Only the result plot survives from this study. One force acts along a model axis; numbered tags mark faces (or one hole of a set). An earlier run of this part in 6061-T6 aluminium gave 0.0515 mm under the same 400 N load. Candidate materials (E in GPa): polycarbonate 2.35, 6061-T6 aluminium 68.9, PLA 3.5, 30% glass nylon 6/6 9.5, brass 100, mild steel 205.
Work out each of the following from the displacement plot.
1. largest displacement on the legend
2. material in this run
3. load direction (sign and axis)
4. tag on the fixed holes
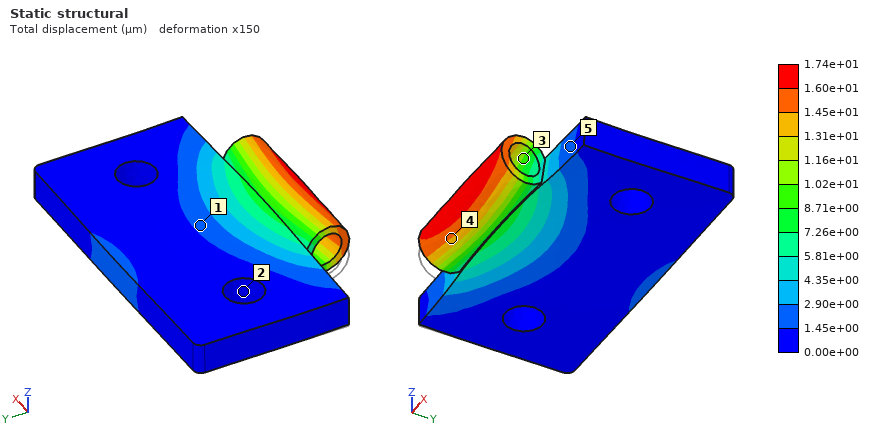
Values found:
1.74e+01 µm
mild steel
+Z
2
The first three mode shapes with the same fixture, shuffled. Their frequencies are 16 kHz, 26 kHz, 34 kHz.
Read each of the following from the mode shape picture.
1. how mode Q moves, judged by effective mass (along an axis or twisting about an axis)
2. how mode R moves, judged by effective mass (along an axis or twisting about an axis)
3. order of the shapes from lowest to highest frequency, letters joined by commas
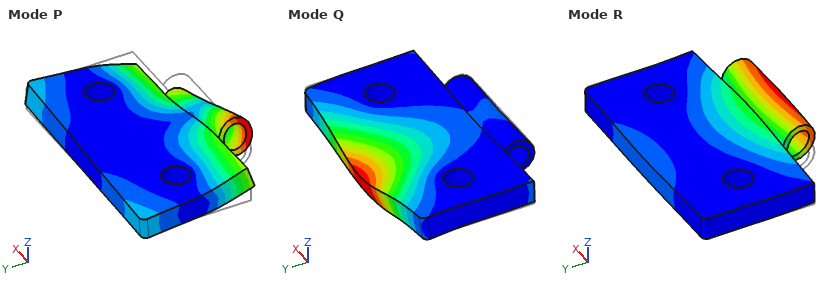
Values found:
along Z
along Z
R, Q, P
